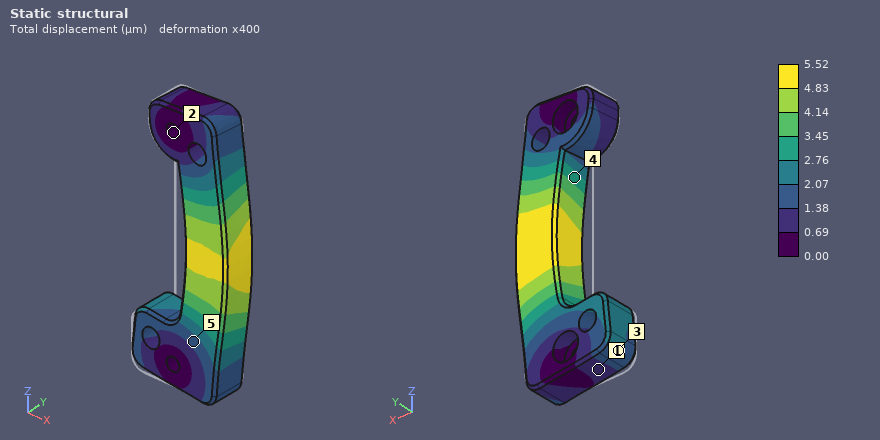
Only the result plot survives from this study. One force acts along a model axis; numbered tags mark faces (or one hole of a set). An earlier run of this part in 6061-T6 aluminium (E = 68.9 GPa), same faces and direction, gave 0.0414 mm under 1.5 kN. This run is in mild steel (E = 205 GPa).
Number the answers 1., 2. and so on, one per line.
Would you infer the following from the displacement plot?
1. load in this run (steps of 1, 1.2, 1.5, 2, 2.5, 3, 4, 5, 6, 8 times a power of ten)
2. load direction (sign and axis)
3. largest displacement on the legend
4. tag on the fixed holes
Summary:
1. 600 N
2. +X
3. 5.52 µm
4. 2
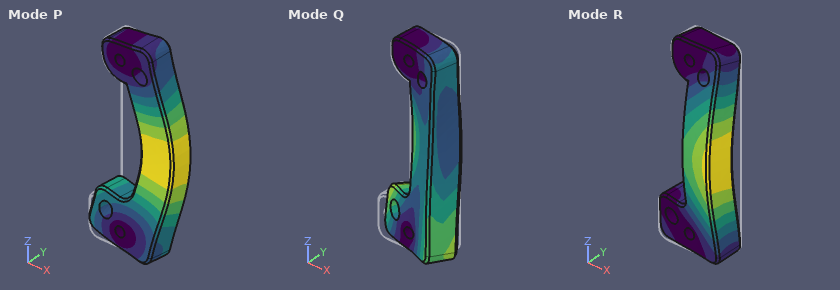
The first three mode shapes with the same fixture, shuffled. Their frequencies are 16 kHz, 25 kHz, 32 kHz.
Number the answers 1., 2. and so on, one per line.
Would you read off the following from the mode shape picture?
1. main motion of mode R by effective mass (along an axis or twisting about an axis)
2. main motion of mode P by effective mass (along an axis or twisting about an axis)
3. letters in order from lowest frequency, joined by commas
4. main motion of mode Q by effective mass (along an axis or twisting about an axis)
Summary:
1. along Y
2. along X
3. R, P, Q
4. twisting about Z
